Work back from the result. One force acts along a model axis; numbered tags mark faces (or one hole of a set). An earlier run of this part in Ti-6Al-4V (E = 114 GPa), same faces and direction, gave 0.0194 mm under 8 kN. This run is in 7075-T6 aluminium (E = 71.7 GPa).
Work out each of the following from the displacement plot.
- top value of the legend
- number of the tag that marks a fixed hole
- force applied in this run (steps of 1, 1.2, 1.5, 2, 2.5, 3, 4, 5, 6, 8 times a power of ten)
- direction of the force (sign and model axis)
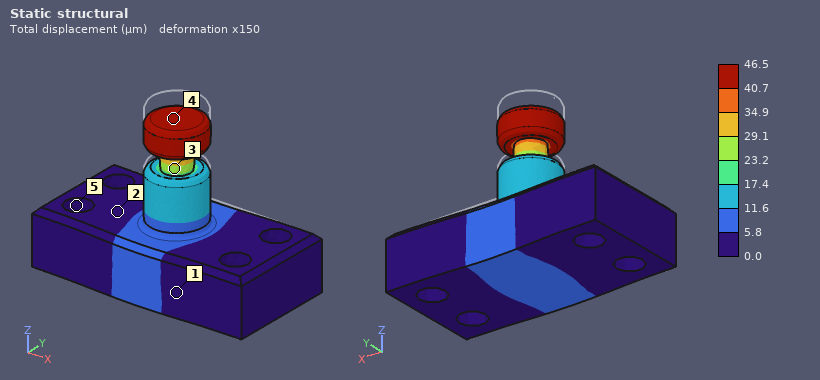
46.5 µm
5
12 kN
-Z
